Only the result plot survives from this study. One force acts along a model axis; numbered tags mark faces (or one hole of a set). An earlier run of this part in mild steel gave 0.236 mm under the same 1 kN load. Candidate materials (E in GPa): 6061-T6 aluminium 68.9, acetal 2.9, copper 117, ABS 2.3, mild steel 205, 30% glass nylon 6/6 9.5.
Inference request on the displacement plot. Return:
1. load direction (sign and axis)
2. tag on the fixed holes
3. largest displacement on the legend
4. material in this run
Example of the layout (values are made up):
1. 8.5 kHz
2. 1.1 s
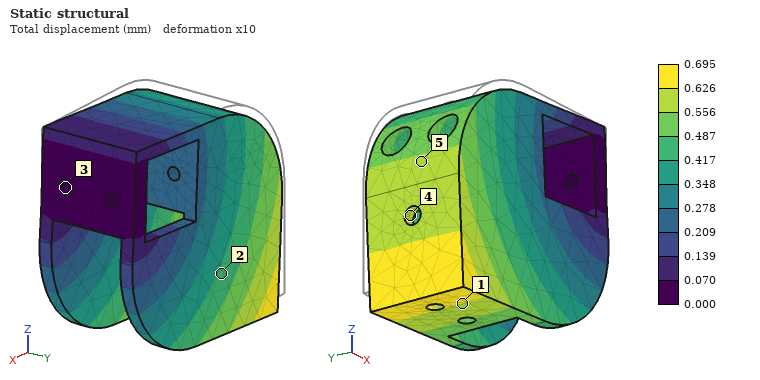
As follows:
1. -Z
2. 3
3. 0.695 mm
4. 6061-T6 aluminium
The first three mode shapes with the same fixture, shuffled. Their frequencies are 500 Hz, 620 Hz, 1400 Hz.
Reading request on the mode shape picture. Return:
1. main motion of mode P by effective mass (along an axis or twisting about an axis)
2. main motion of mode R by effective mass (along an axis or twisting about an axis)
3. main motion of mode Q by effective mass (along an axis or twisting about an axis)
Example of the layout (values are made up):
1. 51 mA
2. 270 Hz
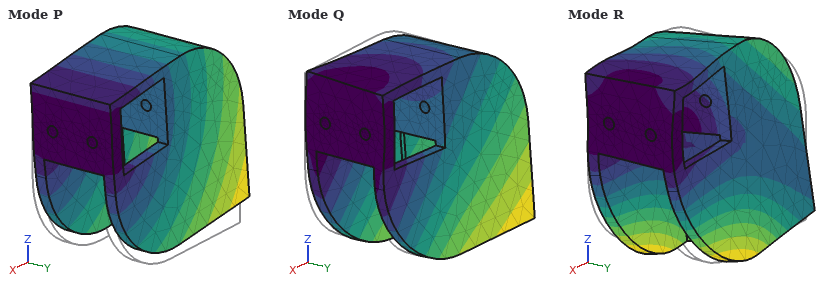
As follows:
1. along Z
2. twisting about X
3. along Y
